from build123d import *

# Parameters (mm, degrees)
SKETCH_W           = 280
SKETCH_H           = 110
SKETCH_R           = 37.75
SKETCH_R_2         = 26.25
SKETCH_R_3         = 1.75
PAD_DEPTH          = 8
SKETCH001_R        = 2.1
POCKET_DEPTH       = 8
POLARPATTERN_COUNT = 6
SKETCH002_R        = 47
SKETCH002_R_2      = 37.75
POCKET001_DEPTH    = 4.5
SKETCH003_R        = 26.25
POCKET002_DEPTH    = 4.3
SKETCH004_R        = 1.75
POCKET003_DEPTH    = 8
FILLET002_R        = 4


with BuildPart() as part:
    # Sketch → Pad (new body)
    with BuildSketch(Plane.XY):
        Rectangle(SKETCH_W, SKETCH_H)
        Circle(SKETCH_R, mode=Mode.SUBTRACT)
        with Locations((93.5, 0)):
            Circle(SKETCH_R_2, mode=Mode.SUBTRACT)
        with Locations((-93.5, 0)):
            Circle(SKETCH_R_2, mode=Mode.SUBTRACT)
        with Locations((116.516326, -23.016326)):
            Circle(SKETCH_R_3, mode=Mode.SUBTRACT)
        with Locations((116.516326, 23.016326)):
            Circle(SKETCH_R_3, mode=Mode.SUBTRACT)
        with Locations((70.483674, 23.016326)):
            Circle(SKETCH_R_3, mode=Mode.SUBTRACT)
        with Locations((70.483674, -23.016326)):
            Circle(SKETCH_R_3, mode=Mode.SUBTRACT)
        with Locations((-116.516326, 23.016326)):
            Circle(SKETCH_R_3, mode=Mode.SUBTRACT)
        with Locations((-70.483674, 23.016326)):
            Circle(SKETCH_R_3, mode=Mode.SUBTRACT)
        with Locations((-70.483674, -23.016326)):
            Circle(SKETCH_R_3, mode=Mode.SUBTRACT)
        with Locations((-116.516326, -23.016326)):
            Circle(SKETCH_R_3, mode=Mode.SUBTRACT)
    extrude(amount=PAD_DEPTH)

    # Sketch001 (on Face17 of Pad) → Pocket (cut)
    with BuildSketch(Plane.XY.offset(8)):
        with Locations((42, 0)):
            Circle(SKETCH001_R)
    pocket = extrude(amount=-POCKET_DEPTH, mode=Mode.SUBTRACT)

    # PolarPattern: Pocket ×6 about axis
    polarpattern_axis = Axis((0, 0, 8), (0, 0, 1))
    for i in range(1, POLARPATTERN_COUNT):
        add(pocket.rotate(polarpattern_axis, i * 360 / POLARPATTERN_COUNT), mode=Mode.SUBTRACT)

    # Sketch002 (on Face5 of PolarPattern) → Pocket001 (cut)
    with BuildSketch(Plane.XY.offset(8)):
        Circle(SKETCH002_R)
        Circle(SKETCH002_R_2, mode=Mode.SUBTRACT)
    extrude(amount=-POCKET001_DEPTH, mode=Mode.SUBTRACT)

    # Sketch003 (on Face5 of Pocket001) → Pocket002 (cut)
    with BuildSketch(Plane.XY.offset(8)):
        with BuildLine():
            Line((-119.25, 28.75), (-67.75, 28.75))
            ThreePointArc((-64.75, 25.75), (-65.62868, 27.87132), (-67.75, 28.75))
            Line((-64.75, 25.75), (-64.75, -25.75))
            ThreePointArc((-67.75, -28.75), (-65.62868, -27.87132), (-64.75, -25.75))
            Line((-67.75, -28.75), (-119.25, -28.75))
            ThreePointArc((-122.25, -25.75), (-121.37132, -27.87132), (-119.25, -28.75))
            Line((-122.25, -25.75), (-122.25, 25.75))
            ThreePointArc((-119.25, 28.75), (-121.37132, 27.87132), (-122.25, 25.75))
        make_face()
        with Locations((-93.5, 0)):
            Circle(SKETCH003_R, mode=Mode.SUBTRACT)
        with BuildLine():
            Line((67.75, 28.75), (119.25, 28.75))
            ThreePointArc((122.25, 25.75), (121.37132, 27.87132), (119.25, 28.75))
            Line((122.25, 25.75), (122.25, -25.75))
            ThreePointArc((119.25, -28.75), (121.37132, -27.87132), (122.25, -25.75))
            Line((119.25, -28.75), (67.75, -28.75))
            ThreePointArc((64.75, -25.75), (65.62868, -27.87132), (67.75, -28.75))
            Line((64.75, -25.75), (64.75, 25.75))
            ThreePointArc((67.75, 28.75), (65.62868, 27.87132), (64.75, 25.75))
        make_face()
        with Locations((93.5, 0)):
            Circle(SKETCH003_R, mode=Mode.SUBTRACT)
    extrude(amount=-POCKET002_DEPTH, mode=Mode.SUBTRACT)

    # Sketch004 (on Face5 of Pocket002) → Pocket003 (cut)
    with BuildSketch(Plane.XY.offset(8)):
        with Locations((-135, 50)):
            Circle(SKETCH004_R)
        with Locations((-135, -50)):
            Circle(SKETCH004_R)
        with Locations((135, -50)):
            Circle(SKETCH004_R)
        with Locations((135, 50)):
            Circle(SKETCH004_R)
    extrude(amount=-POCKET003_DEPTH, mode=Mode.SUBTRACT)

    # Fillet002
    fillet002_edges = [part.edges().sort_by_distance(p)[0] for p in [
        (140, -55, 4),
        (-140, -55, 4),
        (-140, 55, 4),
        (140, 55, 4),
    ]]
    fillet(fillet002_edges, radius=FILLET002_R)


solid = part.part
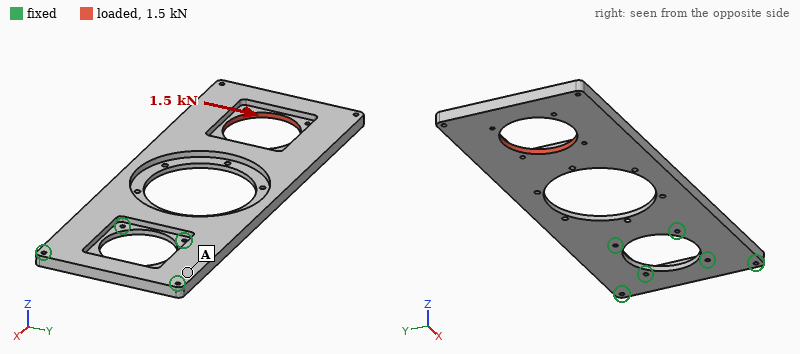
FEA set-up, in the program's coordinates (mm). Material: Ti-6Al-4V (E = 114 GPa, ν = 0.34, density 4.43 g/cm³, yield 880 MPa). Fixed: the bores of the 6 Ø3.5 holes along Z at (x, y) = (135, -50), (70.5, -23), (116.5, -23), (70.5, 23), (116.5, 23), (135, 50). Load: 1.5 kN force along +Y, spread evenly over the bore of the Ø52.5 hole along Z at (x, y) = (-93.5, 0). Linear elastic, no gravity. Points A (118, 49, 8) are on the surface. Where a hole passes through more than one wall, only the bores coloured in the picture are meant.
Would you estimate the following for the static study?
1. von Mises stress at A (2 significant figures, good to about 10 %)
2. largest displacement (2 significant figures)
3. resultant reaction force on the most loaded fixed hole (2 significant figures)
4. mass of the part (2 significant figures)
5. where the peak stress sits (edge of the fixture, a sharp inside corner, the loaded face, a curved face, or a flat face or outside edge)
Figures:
8.3 MPa
0.17 mm
1.6 kN
680 g
a curved face
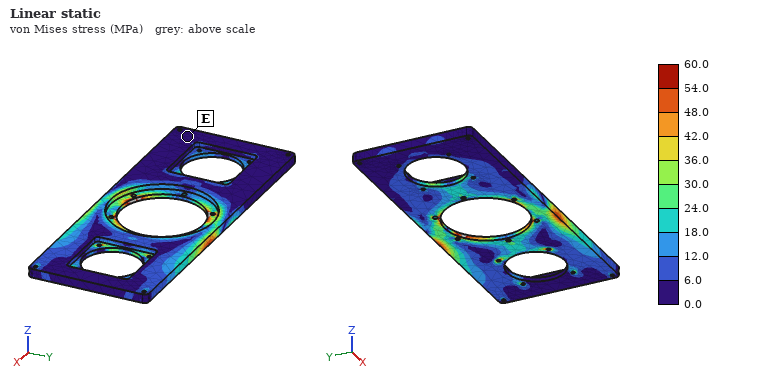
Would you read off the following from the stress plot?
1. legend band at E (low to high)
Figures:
0.0 to 6.0 MPa
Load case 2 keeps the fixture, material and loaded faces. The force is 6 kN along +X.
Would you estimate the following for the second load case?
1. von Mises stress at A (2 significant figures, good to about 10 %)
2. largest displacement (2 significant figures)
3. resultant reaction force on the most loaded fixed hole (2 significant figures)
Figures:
7.2 MPa
1.1 mm
1.6 kN
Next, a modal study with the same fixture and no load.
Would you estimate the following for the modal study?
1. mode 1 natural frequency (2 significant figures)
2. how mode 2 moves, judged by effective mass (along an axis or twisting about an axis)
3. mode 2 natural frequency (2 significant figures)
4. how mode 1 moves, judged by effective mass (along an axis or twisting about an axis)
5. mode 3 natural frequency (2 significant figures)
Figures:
100 Hz
twisting about X
380 Hz
along Z
720 Hz
